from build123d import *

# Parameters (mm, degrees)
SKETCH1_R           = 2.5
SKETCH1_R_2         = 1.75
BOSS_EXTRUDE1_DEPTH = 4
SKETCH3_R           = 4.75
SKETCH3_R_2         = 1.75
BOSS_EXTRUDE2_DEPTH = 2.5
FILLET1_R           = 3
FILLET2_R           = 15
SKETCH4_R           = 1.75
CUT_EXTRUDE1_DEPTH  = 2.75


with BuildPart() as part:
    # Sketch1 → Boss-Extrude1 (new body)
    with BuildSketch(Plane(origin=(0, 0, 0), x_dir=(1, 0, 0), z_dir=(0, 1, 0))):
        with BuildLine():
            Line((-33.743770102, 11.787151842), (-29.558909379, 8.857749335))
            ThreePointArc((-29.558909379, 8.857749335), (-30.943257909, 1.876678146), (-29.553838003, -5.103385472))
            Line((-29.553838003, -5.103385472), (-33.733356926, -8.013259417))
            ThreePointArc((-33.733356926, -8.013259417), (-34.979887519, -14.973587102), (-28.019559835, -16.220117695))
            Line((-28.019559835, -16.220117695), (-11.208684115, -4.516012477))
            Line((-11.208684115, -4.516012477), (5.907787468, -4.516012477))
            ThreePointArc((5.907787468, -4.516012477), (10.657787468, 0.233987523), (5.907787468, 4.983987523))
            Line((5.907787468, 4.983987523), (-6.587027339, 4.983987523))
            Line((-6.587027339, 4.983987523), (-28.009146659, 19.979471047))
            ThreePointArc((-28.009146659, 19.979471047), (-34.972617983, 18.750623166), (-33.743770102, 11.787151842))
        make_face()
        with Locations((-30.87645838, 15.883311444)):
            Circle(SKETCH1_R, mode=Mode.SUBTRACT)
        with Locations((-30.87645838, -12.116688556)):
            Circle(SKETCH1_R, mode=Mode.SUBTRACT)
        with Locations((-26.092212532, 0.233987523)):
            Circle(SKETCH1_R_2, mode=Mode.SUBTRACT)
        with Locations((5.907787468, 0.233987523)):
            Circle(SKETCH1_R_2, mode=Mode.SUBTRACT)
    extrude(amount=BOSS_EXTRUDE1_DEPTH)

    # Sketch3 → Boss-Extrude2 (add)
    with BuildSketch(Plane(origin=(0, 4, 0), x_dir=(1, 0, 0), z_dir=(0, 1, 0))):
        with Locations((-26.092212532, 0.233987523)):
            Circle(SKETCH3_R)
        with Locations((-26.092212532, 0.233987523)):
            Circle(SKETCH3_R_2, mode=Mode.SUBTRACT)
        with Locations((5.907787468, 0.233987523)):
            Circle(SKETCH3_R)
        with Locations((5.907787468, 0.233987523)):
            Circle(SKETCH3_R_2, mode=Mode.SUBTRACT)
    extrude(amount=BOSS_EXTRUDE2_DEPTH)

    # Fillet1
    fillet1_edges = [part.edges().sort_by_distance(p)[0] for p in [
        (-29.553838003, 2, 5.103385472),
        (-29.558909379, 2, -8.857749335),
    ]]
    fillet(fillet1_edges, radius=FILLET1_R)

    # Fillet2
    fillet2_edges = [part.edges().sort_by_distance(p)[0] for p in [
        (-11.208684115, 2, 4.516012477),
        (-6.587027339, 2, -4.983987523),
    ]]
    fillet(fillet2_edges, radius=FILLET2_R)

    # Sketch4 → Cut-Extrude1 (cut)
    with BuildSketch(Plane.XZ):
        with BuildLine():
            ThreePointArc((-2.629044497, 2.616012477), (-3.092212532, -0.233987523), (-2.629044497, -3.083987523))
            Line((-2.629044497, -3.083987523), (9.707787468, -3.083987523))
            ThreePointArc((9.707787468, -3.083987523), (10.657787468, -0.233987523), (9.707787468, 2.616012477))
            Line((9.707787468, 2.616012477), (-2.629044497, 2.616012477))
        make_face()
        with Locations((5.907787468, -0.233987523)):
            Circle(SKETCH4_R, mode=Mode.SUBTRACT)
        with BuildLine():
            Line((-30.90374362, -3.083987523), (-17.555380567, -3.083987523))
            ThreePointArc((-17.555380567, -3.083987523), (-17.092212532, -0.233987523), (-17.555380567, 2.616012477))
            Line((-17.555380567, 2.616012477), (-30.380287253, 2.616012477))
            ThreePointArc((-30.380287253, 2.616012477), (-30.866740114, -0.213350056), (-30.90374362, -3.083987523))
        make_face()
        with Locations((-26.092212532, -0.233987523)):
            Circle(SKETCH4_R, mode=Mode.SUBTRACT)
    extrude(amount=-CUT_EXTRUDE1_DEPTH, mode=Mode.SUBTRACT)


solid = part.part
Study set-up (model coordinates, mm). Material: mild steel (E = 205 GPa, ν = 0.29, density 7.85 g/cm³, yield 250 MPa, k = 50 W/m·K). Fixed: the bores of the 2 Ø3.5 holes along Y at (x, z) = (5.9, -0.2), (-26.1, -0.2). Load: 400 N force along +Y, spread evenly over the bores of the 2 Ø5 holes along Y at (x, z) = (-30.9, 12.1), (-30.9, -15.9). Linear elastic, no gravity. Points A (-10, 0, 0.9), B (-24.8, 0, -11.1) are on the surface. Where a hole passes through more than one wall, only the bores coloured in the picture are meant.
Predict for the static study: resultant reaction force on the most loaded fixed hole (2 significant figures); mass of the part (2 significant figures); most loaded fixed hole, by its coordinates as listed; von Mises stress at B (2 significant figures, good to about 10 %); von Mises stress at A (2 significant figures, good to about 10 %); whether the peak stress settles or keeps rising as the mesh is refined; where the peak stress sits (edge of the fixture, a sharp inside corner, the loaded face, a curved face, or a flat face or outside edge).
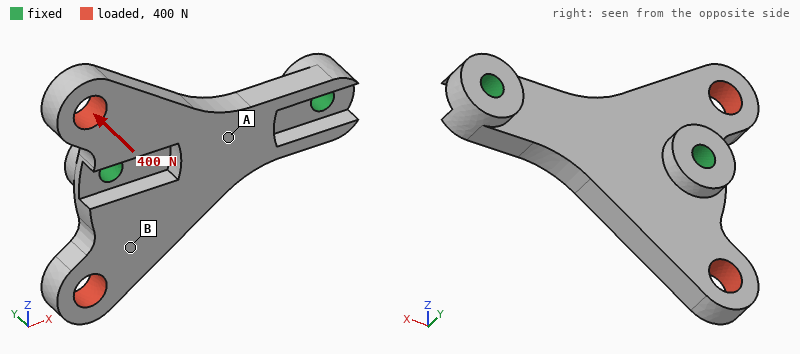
440 N
23 g
(-26.1, -0.2)
48 MPa
15 MPa
keeps rising
edge of the fixture
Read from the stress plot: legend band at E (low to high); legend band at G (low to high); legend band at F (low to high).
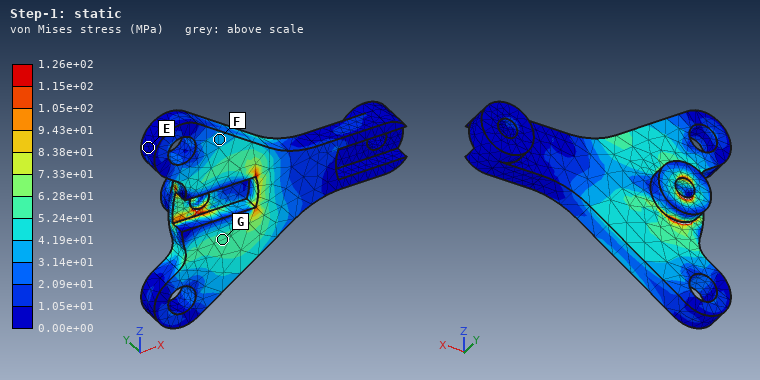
0.00e+00 to 1.05e+01 MPa
5.24e+01 to 6.28e+01 MPa
3.14e+01 to 4.19e+01 MPa
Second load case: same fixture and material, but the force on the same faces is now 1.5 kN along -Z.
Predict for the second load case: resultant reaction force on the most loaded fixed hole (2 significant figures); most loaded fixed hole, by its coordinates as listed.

1.7 kN
(-26.1, -0.2)
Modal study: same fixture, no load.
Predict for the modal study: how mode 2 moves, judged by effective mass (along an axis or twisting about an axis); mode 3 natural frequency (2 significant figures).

along Y
15 kHz
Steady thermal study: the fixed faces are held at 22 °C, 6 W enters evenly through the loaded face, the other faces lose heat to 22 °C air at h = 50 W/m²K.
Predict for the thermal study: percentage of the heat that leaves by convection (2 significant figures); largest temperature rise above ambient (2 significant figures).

17 %
27 K
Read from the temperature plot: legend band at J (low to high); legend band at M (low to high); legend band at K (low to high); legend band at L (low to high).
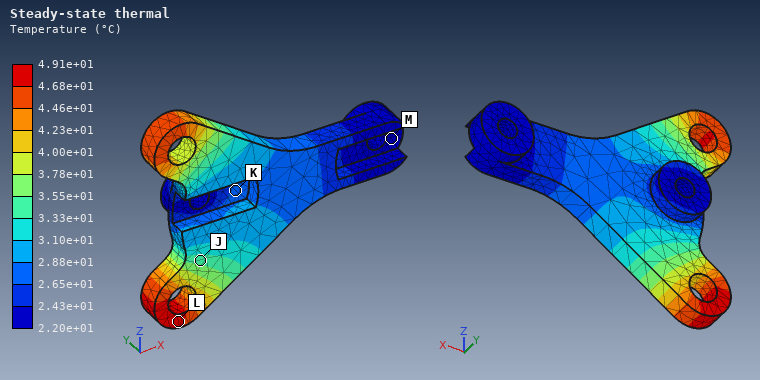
3.33e+01 to 3.55e+01 °C
2.20e+01 to 2.43e+01 °C
2.65e+01 to 2.88e+01 °C
4.68e+01 to 4.91e+01 °C
